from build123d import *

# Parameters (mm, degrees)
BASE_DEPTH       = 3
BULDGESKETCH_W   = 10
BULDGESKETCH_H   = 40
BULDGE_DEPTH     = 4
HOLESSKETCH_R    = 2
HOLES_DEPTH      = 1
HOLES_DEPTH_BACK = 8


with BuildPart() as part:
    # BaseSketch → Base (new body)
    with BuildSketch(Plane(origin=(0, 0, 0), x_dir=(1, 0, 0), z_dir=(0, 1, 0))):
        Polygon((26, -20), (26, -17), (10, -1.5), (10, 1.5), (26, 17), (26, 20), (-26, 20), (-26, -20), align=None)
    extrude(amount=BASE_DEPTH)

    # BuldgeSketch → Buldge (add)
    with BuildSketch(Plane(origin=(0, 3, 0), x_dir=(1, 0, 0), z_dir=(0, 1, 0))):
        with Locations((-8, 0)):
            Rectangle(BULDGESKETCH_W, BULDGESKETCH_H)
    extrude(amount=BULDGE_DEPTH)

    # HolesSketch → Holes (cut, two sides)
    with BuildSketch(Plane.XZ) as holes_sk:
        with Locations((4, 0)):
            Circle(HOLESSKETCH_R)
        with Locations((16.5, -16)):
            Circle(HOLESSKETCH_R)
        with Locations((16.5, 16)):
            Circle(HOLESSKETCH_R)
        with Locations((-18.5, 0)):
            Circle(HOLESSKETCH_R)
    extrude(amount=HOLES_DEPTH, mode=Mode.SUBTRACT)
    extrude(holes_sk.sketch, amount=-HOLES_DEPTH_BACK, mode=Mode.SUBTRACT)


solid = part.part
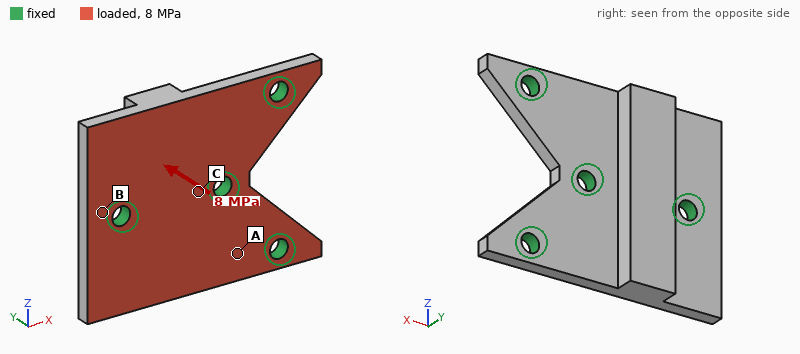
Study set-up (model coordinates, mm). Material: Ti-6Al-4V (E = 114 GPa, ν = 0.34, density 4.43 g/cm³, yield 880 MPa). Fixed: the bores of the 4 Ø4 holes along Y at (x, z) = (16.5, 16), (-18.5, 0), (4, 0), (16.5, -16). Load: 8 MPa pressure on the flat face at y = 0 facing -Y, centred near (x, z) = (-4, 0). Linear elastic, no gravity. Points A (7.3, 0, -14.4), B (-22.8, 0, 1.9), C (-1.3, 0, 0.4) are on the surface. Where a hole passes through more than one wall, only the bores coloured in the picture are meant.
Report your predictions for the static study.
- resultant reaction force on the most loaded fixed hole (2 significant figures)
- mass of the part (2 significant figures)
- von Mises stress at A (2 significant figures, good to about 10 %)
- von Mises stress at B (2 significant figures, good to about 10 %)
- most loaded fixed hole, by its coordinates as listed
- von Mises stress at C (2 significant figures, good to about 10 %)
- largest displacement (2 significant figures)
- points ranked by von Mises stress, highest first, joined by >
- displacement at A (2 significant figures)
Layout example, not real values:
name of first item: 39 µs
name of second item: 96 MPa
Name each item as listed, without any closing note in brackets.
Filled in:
resultant reaction force on the most loaded fixed hole: 6.5 kN
mass of the part: 30 g
von Mises stress at A: 100 MPa
von Mises stress at B: 310 MPa
most loaded fixed hole, by its coordinates as listed: (-18.5, 0)
von Mises stress at C: 200 MPa
largest displacement: 0.21 mm
points ranked by von Mises stress, highest first, joined by >: B > C > A
displacement at A: 0.040 mm
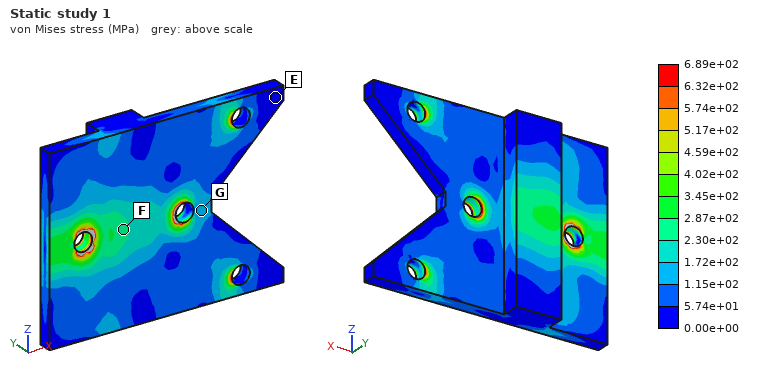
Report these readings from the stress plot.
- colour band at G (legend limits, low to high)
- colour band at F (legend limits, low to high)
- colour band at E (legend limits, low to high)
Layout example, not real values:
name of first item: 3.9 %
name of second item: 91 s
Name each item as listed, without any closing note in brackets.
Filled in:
colour band at G: 1.15e+02 to 1.72e+02 MPa
colour band at F: 2.30e+02 to 2.87e+02 MPa
colour band at E: 0.00e+00 to 5.74e+01 MPa
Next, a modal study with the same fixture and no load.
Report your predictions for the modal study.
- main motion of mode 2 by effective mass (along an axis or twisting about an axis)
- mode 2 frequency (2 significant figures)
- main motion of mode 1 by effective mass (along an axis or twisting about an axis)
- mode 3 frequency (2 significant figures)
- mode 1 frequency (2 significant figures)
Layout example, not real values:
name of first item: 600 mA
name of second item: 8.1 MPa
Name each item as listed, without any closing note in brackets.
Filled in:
main motion of mode 2 by effective mass: along Y
mode 2 frequency: 11 kHz
main motion of mode 1 by effective mass: twisting about X
mode 3 frequency: 16 kHz
mode 1 frequency: 6800 Hz
